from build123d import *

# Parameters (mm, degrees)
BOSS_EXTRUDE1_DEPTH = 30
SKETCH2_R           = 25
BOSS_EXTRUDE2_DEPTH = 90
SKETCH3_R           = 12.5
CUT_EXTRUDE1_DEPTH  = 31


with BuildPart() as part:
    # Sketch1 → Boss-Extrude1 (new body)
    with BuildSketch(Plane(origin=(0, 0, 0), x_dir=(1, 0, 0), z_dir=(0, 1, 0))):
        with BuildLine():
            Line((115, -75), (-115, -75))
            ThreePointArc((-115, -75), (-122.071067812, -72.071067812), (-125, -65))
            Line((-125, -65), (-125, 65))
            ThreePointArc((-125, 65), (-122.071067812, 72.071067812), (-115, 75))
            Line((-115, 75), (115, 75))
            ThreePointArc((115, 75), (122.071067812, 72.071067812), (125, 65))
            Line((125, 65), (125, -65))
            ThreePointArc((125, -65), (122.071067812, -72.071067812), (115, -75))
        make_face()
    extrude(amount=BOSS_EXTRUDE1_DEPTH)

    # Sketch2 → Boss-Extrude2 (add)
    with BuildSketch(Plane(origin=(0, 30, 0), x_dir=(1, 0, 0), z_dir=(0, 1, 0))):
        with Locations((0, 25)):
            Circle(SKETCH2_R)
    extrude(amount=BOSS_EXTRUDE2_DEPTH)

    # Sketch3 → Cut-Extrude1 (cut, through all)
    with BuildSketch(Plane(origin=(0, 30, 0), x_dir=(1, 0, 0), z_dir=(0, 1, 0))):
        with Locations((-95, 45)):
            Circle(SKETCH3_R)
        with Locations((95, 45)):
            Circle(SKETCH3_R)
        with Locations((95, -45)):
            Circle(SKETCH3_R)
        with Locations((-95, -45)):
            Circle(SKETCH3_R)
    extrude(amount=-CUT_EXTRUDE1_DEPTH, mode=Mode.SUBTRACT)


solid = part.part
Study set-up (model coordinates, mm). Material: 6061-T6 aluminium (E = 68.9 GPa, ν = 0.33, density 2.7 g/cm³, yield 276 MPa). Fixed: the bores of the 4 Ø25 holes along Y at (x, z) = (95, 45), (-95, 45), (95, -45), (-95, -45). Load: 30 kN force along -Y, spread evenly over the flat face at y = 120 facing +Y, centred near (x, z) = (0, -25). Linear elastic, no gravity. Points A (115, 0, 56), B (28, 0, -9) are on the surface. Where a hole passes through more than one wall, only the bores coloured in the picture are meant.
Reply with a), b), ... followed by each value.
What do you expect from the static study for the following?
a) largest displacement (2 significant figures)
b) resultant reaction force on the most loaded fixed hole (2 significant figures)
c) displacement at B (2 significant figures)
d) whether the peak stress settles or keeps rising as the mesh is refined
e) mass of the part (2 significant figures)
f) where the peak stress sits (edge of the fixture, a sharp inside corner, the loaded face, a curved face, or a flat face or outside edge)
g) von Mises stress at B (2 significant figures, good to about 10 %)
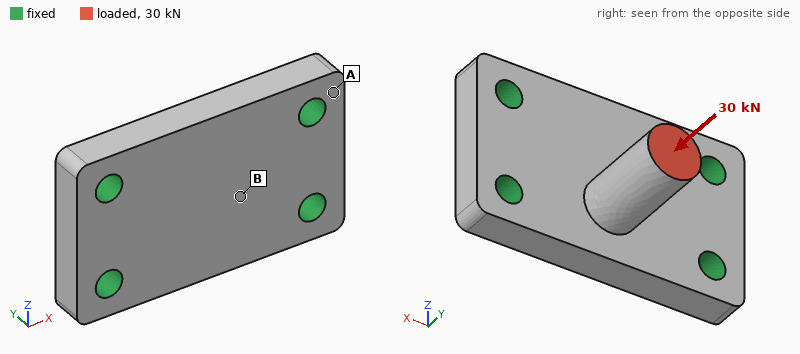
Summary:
a) 84 µm
b) 11 kN
c) 43 µm
d) keeps rising
e) 3.3 kg
f) edge of the fixture
g) 18 MPa
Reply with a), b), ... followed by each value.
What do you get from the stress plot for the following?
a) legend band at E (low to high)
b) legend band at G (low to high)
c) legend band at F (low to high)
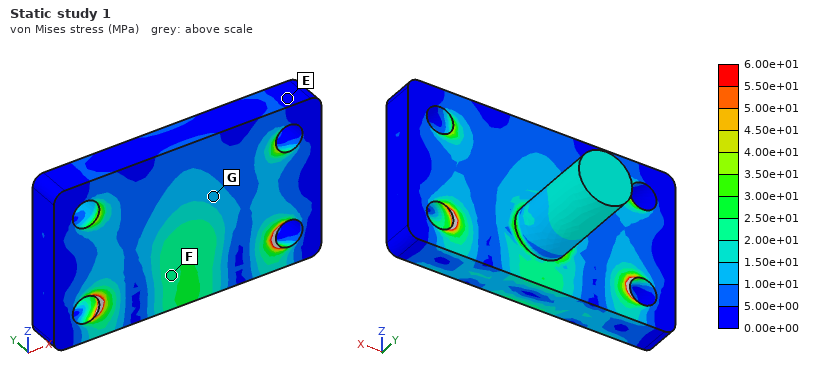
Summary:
a) 0.00e+00 to 5.00e+00 MPa
b) 1.00e+01 to 1.50e+01 MPa
c) 2.00e+01 to 2.50e+01 MPa
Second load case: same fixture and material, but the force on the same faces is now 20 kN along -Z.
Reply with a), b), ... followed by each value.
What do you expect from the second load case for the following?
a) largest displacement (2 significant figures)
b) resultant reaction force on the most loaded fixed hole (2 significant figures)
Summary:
a) 0.57 mm
b) 12 kN
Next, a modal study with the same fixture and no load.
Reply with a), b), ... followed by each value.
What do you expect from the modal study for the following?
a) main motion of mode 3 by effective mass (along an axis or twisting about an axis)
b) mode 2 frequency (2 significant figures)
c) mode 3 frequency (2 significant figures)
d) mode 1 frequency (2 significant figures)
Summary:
a) along Y
b) 2700 Hz
c) 3400 Hz
d) 2300 Hz
